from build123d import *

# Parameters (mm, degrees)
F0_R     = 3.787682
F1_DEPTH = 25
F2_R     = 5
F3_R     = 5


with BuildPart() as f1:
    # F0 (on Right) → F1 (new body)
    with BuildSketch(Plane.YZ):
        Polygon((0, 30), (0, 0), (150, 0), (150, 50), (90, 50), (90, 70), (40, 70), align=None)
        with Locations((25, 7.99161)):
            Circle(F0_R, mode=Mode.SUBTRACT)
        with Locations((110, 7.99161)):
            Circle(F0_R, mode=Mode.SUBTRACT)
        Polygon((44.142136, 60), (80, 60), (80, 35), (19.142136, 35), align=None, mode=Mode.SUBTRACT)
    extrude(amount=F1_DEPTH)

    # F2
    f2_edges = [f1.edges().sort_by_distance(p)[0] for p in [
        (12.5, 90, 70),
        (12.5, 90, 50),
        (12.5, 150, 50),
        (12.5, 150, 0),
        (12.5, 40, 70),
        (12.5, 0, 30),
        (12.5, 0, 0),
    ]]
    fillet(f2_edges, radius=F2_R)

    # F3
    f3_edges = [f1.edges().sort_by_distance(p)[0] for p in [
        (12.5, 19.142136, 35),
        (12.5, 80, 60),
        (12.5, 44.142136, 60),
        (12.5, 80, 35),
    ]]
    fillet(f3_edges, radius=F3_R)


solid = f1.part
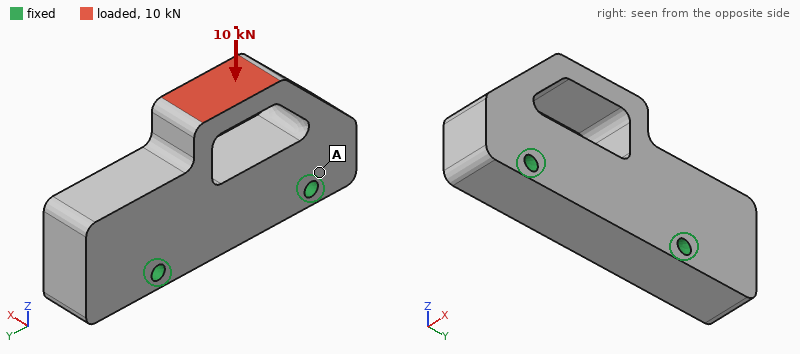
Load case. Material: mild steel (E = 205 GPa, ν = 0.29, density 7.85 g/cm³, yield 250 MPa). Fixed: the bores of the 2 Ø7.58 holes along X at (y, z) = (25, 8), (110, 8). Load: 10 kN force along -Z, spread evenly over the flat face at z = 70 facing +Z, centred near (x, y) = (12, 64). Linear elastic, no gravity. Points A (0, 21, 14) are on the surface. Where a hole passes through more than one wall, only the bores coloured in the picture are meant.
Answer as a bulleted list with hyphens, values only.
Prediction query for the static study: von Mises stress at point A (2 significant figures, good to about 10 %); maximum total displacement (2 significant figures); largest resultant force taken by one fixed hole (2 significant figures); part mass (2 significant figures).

- 14 MPa
- 20 µm
- 5.3 kN
- 1.4 kg
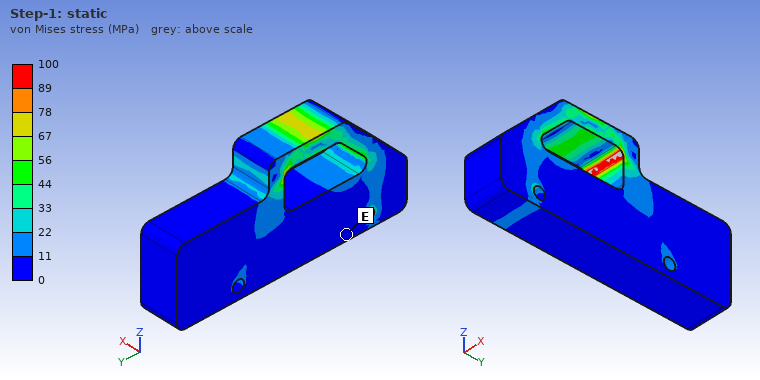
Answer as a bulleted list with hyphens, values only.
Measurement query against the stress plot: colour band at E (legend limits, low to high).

- 0 to 11 MPa
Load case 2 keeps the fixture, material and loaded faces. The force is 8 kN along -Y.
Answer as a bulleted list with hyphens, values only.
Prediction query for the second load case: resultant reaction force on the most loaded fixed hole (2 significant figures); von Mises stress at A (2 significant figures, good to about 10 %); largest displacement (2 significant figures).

- 6.8 kN
- 13 MPa
- 18 µm
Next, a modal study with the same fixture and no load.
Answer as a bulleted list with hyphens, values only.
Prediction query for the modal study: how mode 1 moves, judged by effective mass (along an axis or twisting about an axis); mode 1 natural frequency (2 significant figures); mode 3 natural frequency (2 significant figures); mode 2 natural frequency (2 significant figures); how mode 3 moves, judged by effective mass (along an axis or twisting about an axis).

- along X
- 4500 Hz
- 7100 Hz
- 6500 Hz
- along Y
